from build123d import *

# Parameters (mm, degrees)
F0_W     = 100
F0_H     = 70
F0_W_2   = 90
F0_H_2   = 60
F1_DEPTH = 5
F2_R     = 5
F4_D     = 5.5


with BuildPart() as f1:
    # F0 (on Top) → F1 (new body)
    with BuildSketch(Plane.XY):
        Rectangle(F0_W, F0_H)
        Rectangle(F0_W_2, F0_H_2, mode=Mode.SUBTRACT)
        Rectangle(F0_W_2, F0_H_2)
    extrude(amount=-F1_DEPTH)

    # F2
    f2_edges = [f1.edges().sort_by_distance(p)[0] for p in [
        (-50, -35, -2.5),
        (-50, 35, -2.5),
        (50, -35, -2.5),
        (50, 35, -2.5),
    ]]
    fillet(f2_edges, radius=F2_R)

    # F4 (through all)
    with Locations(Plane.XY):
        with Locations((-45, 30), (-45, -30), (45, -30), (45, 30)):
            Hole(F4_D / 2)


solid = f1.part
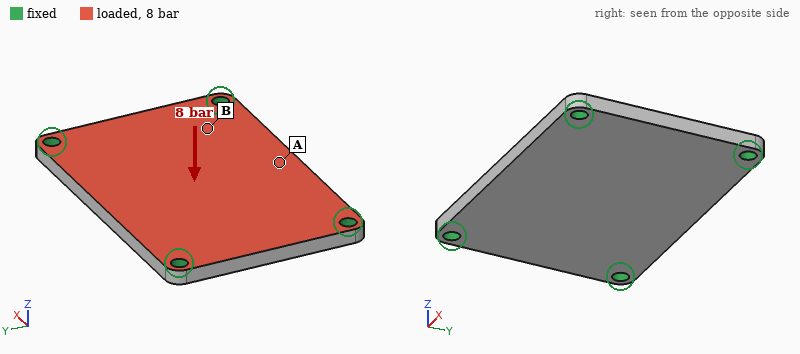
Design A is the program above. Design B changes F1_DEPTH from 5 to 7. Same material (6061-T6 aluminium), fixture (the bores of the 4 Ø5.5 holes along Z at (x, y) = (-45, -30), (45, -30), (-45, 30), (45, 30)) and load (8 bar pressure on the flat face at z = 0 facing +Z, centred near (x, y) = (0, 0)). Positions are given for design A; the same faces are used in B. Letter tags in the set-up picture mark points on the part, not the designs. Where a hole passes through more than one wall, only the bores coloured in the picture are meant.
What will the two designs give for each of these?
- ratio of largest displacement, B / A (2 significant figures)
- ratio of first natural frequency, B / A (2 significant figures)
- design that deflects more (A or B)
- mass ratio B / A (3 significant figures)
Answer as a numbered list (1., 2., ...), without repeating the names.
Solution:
1. 0.39
2. 1.3
3. A
4. 1.40
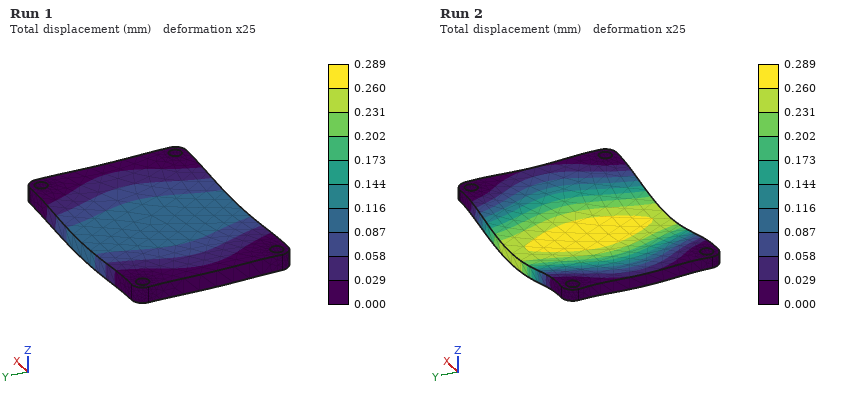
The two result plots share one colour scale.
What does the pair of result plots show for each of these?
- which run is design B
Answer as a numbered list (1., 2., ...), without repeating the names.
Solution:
1. Run 1
